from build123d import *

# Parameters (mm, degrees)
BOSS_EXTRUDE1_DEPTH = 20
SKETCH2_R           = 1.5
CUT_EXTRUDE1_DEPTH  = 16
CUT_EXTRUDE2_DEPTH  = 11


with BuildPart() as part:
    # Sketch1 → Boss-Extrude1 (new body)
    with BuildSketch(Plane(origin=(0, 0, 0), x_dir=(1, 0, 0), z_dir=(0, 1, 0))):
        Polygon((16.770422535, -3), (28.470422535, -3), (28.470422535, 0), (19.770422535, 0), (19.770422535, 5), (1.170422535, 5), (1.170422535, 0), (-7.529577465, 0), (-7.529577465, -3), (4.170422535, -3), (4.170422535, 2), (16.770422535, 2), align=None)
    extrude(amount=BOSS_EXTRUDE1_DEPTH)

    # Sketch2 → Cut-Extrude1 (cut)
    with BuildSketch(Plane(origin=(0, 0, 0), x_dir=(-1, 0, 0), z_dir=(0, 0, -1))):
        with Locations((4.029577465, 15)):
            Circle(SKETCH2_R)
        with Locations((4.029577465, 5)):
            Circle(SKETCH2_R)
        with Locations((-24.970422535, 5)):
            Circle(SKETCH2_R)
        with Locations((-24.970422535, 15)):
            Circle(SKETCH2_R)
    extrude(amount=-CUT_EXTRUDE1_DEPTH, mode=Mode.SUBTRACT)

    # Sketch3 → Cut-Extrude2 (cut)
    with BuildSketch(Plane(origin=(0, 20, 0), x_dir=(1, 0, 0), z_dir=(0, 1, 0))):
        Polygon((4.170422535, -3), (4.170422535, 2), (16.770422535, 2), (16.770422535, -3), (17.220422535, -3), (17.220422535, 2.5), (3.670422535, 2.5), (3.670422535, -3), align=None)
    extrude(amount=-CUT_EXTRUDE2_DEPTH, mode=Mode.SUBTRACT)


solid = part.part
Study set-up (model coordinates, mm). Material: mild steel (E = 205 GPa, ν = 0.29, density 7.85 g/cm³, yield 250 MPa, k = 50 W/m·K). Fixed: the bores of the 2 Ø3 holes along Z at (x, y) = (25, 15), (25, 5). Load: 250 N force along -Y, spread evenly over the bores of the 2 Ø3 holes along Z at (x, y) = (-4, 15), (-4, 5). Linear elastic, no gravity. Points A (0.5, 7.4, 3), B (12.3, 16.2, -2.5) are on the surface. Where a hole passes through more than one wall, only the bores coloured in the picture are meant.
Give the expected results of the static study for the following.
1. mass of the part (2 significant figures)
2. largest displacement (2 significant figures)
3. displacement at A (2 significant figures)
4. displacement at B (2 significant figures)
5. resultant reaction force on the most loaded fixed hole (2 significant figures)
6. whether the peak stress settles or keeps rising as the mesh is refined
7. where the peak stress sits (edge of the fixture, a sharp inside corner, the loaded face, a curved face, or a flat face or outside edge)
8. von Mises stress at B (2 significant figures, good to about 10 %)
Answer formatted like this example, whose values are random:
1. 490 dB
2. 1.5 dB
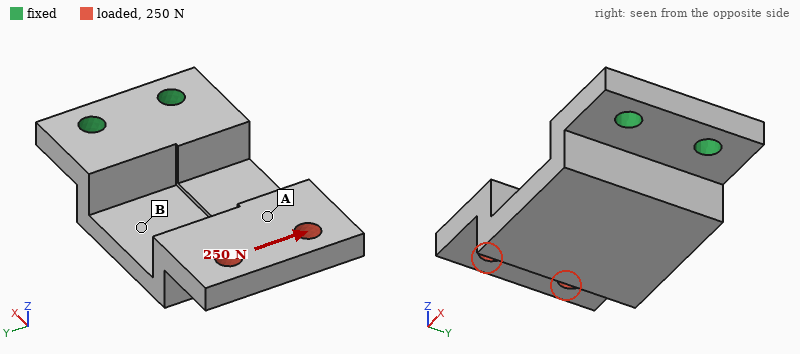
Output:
1. 20 g
2. 57 µm
3. 38 µm
4. 14 µm
5. 600 N
6. keeps rising
7. a sharp inside corner
8. 65 MPa
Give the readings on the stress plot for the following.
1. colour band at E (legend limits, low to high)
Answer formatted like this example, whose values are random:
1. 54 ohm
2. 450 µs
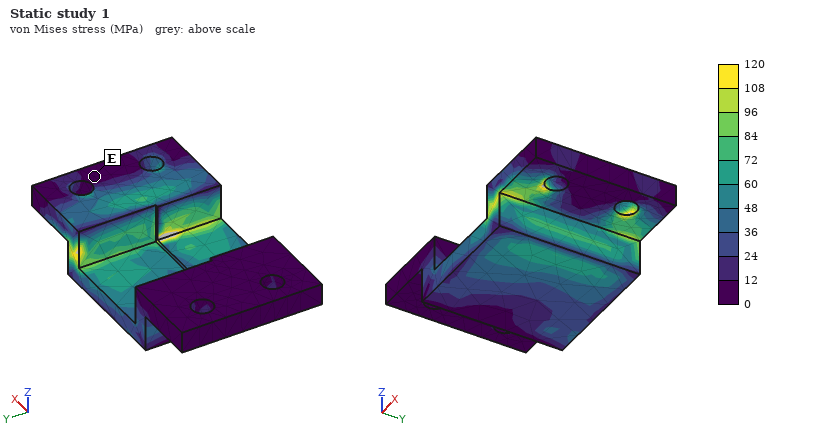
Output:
1. 0 to 12 MPa
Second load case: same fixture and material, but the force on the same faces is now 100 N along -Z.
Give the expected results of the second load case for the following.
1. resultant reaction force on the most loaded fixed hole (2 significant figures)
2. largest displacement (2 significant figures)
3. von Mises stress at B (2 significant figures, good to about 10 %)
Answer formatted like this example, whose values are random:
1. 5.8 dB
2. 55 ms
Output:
1. 51 N
2. 0.14 mm
3. 56 MPa
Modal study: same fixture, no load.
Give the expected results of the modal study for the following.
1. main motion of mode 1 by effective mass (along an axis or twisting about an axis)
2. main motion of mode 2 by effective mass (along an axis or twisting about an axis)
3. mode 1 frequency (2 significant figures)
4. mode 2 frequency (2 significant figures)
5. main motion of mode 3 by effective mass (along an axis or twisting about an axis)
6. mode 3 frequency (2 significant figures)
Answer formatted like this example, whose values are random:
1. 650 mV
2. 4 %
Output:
1. along Z
2. along Y
3. 1900 Hz
4. 4700 Hz
5. along X
6. 8000 Hz
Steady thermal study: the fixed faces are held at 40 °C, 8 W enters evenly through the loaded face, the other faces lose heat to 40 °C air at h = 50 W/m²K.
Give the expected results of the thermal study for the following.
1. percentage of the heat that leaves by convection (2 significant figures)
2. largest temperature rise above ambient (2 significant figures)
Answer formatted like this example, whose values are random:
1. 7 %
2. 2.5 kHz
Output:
1. 42 %
2. 71 K
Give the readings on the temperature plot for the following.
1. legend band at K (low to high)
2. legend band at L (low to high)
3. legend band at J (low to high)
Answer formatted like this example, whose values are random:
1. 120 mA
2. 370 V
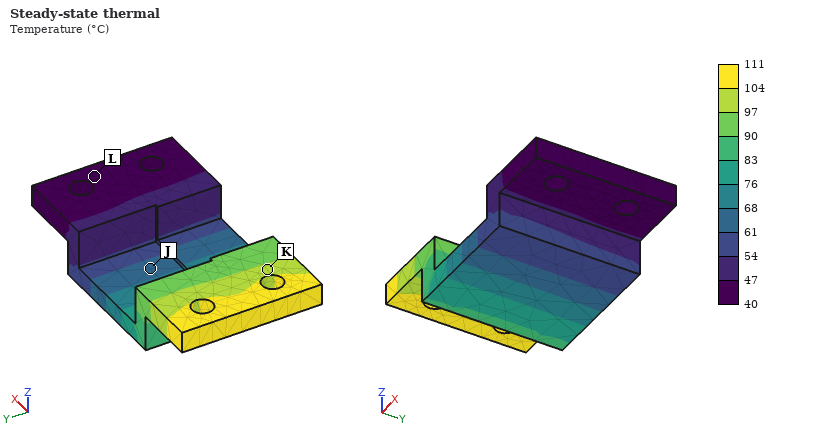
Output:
1. 97 to 104 °C
2. 40 to 47 °C
3. 61 to 68 °C
